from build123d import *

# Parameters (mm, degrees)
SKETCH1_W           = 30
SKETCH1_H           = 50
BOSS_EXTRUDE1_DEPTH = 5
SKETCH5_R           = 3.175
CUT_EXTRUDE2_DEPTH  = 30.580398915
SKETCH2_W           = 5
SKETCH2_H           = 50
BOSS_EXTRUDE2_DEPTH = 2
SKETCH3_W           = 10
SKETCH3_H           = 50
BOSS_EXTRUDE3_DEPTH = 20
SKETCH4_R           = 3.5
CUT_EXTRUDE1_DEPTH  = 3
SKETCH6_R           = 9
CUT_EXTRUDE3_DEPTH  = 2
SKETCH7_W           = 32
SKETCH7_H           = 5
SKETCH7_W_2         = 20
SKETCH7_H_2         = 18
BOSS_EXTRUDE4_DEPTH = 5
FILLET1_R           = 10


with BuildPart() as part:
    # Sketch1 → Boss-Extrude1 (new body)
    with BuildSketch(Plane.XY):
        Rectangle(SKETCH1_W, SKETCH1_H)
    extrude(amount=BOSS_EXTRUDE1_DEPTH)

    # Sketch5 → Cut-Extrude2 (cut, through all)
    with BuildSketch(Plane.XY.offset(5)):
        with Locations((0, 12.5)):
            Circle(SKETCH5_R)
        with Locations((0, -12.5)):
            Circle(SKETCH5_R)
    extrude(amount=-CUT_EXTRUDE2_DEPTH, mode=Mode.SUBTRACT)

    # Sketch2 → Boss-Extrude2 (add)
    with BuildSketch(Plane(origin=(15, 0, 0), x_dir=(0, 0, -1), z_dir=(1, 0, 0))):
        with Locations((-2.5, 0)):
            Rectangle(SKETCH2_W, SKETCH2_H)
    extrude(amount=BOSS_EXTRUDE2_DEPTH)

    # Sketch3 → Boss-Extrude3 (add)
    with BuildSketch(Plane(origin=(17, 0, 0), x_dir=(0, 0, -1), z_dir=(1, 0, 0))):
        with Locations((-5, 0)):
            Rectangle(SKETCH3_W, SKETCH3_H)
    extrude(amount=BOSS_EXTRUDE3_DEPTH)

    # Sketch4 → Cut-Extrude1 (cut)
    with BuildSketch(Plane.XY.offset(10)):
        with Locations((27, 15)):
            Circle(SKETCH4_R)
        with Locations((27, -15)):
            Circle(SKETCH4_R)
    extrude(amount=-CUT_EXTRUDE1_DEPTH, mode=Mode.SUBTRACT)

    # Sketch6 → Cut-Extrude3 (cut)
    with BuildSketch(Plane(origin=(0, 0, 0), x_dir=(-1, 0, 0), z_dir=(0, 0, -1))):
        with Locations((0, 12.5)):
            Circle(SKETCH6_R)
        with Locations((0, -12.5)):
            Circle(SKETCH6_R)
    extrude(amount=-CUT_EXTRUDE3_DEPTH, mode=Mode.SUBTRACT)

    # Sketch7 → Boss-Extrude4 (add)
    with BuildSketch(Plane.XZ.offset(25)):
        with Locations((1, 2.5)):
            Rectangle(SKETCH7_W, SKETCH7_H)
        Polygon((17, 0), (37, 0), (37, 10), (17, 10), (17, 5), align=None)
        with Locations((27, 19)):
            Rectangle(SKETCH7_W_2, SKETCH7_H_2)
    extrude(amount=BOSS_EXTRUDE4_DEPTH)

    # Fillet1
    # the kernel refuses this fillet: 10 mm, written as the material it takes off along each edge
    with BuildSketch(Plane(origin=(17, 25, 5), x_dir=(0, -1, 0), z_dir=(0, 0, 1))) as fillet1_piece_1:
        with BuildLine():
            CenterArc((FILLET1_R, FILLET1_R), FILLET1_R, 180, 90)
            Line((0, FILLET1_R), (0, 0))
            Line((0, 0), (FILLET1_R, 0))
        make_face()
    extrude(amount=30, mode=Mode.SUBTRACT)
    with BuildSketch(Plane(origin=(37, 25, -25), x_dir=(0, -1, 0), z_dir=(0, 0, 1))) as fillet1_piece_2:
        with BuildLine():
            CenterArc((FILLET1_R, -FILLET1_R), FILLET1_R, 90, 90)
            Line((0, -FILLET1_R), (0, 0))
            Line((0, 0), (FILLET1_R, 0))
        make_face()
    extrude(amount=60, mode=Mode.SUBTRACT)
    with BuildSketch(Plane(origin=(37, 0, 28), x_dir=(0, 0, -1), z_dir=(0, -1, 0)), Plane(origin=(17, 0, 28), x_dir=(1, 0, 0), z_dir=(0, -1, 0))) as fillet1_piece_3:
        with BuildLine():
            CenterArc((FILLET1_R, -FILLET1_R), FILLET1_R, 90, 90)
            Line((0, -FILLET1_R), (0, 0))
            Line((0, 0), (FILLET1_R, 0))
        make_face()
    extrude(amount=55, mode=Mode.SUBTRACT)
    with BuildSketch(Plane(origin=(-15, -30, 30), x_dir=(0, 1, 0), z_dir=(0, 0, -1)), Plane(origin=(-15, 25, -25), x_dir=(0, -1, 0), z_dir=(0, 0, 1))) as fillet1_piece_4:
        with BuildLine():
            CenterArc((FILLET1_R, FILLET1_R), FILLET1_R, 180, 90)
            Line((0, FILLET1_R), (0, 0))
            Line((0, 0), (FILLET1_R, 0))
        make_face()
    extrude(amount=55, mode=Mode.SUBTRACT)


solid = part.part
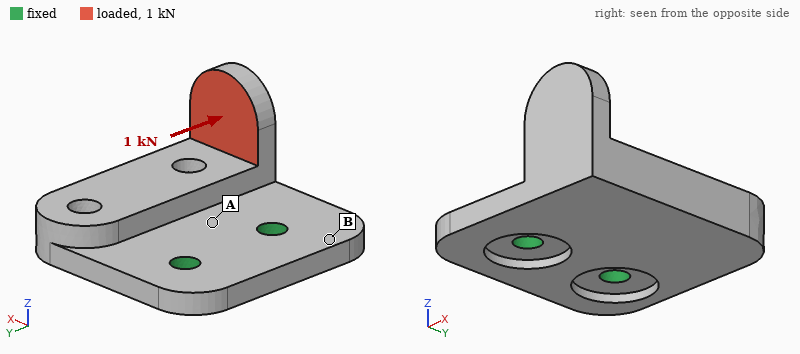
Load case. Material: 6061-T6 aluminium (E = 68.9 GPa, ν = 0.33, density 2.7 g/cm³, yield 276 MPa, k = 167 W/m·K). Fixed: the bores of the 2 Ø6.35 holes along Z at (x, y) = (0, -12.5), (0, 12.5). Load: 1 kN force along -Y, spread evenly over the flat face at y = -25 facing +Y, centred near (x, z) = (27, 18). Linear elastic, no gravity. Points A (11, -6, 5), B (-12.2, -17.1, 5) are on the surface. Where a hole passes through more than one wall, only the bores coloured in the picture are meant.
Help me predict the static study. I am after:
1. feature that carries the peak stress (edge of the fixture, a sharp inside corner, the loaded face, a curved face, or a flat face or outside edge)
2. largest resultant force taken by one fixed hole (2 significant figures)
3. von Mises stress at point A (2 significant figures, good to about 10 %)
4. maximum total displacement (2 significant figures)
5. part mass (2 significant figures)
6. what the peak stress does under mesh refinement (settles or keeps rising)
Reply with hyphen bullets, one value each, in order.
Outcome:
- edge of the fixture
- 1.2 kN
- 44 MPa
- 0.23 mm
- 52 g
- keeps rising
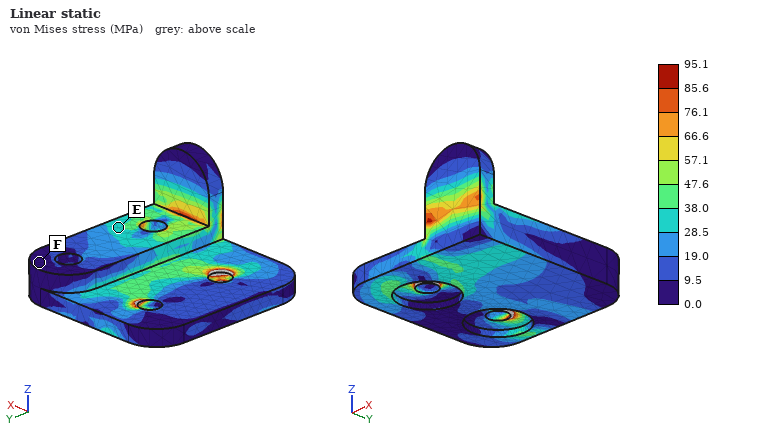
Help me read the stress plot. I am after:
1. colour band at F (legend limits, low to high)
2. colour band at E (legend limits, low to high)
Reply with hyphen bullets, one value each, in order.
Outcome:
- 0.0 to 9.5 MPa
- 28.5 to 38.0 MPa
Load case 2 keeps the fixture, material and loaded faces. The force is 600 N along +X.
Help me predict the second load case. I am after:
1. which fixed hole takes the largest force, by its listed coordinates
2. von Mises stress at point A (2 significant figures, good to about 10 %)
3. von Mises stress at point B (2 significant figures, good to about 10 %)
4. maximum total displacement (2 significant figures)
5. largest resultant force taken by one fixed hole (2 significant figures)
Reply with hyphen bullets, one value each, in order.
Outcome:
- (0, -12.5)
- 44 MPa
- 10 MPa
- 0.27 mm
- 840 N
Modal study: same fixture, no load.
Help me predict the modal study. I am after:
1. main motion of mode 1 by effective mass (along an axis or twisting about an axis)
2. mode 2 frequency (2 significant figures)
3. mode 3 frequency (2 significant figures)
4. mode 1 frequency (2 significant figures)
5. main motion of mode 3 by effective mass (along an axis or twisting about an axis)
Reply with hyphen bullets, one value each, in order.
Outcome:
- along Z
- 3500 Hz
- 7300 Hz
- 1400 Hz
- along Y
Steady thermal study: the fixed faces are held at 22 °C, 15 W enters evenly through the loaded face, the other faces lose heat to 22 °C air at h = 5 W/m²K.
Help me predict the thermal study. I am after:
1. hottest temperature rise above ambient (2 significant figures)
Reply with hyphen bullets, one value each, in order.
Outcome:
- 25 K
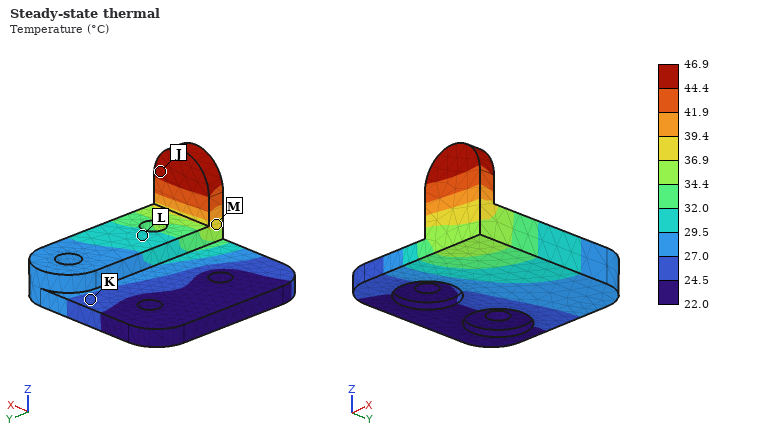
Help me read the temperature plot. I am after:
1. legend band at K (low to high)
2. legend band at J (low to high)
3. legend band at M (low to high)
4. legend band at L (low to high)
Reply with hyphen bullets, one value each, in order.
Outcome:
- 24.5 to 27.0 °C
- 44.4 to 46.9 °C
- 36.9 to 39.4 °C
- 29.5 to 32.0 °C
